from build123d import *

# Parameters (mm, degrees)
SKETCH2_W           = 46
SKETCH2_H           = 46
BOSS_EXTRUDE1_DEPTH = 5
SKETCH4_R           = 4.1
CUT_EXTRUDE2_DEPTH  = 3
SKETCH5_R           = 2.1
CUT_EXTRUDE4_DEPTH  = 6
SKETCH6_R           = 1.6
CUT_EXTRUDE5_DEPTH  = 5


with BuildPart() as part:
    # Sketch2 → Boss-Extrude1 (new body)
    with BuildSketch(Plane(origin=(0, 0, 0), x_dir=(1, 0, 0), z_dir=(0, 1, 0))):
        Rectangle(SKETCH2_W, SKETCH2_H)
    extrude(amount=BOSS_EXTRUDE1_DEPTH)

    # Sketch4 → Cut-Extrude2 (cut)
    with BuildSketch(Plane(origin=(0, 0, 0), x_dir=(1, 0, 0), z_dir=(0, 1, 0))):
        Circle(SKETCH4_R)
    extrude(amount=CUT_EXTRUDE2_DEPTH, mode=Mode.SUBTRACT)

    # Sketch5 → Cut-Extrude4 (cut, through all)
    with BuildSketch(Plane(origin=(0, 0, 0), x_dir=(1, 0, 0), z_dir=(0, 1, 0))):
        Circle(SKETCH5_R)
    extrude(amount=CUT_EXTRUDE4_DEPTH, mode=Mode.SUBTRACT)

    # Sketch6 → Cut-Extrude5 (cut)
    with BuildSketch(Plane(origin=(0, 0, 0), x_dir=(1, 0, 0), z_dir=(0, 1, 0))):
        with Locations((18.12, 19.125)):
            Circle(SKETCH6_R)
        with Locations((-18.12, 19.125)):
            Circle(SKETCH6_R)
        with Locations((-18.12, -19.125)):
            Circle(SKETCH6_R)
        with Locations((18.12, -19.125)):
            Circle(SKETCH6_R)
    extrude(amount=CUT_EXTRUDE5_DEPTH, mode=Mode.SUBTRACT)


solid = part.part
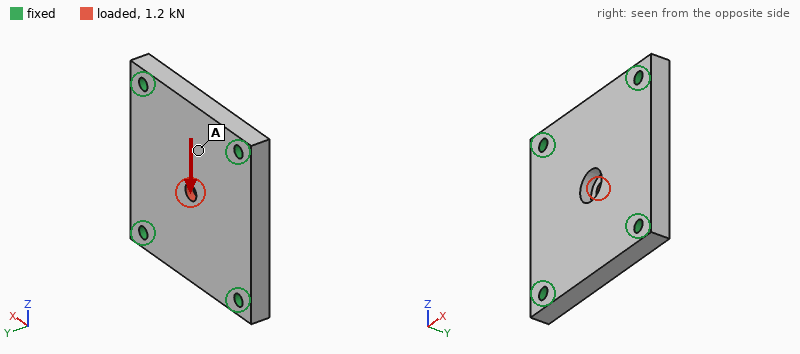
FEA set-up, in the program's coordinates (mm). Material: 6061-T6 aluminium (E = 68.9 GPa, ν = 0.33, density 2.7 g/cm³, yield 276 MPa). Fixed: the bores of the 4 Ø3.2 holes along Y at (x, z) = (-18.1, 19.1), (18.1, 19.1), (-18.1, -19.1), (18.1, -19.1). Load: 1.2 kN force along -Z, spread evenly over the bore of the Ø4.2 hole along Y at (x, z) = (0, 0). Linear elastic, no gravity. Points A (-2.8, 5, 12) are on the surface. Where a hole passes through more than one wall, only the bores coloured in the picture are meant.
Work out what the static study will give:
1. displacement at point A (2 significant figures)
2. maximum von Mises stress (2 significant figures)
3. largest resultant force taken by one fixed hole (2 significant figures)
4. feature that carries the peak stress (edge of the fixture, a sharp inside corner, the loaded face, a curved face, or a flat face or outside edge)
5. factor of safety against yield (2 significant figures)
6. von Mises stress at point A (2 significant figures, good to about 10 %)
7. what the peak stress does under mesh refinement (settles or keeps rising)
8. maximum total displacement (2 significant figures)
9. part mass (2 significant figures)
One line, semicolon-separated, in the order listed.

2.2 µm; 82 MPa; 340 N; the loaded face; 3.4; 6.4 MPa; settles; 5.3 µm; 28 g
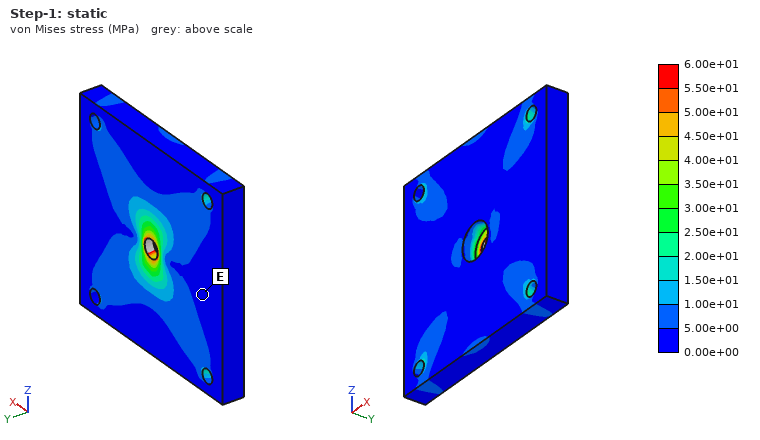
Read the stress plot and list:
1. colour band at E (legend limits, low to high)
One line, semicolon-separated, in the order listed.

0.00e+00 to 5.00e+00 MPa
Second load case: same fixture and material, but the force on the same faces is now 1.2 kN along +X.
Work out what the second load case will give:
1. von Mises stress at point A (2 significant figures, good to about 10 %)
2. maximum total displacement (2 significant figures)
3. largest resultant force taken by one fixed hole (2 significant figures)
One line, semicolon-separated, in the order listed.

5.6 MPa; 5.4 µm; 340 N
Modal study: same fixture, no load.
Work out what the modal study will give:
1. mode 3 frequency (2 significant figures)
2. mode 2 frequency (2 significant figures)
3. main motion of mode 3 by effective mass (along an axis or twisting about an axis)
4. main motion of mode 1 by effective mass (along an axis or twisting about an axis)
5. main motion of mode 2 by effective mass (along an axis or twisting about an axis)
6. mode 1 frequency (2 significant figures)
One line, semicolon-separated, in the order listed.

19 kHz; 18 kHz; twisting about X; along Y; twisting about Z; 12 kHz
